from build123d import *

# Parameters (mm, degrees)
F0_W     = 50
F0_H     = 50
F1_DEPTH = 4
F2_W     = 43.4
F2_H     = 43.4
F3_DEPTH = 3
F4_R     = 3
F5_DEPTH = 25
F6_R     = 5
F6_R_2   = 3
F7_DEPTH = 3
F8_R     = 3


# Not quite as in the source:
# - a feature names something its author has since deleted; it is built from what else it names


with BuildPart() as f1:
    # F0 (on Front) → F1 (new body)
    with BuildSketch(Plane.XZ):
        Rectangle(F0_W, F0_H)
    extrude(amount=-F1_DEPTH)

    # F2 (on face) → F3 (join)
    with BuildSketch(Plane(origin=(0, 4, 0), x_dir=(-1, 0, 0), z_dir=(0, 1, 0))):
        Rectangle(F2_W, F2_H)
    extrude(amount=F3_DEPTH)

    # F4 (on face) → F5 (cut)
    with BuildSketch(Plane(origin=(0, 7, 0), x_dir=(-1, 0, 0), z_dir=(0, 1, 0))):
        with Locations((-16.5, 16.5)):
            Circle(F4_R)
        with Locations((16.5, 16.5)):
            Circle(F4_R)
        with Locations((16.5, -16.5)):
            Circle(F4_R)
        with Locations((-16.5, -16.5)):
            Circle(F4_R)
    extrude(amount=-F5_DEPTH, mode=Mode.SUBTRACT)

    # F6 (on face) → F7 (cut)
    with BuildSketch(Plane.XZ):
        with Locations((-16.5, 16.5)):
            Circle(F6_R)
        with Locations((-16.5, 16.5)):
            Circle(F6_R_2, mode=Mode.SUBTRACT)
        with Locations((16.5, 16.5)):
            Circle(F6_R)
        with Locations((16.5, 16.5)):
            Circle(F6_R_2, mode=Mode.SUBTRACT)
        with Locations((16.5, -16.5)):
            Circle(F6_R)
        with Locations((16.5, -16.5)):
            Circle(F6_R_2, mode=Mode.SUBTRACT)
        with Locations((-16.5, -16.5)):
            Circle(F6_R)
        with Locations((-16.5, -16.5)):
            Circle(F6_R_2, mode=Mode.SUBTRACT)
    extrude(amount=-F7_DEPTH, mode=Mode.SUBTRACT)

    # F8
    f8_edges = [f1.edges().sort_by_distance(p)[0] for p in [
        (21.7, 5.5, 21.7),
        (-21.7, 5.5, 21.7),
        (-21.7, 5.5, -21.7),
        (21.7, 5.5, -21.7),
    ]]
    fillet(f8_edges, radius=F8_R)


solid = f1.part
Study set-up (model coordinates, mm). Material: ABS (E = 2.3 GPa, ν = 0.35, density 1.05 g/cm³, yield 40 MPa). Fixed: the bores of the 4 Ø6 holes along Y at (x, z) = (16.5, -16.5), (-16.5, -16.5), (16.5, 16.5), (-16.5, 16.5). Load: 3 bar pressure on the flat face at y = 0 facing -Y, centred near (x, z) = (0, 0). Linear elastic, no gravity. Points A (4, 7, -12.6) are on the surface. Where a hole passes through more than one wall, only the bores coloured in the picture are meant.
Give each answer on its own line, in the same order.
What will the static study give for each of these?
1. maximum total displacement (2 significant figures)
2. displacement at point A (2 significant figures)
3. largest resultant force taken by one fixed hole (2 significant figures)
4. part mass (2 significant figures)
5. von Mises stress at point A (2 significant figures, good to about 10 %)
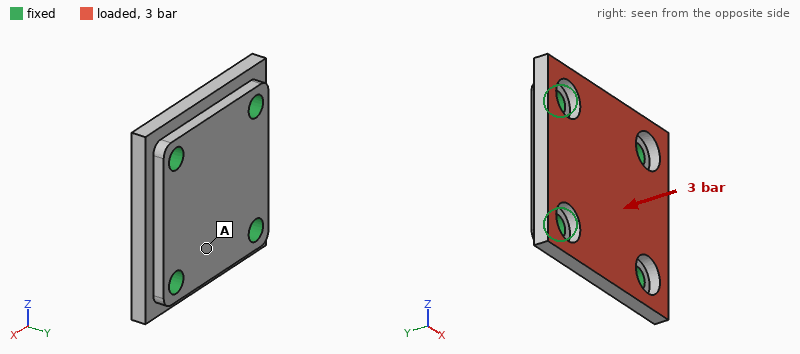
45 µm
32 µm
170 N
15 g
1.5 MPa
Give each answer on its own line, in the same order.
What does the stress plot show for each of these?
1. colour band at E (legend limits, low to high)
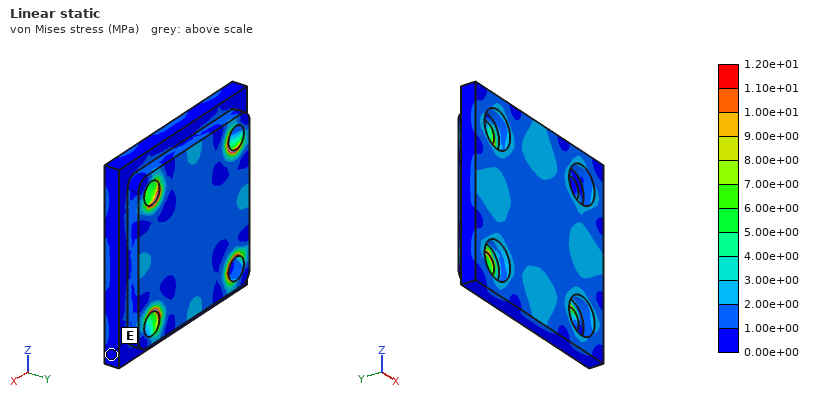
0.00e+00 to 1.00e+00 MPa
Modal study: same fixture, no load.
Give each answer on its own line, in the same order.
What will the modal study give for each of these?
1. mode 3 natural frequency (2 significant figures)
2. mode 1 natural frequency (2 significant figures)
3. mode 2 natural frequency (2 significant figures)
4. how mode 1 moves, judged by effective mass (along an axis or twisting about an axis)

7400 Hz
5500 Hz
7200 Hz
along Y
